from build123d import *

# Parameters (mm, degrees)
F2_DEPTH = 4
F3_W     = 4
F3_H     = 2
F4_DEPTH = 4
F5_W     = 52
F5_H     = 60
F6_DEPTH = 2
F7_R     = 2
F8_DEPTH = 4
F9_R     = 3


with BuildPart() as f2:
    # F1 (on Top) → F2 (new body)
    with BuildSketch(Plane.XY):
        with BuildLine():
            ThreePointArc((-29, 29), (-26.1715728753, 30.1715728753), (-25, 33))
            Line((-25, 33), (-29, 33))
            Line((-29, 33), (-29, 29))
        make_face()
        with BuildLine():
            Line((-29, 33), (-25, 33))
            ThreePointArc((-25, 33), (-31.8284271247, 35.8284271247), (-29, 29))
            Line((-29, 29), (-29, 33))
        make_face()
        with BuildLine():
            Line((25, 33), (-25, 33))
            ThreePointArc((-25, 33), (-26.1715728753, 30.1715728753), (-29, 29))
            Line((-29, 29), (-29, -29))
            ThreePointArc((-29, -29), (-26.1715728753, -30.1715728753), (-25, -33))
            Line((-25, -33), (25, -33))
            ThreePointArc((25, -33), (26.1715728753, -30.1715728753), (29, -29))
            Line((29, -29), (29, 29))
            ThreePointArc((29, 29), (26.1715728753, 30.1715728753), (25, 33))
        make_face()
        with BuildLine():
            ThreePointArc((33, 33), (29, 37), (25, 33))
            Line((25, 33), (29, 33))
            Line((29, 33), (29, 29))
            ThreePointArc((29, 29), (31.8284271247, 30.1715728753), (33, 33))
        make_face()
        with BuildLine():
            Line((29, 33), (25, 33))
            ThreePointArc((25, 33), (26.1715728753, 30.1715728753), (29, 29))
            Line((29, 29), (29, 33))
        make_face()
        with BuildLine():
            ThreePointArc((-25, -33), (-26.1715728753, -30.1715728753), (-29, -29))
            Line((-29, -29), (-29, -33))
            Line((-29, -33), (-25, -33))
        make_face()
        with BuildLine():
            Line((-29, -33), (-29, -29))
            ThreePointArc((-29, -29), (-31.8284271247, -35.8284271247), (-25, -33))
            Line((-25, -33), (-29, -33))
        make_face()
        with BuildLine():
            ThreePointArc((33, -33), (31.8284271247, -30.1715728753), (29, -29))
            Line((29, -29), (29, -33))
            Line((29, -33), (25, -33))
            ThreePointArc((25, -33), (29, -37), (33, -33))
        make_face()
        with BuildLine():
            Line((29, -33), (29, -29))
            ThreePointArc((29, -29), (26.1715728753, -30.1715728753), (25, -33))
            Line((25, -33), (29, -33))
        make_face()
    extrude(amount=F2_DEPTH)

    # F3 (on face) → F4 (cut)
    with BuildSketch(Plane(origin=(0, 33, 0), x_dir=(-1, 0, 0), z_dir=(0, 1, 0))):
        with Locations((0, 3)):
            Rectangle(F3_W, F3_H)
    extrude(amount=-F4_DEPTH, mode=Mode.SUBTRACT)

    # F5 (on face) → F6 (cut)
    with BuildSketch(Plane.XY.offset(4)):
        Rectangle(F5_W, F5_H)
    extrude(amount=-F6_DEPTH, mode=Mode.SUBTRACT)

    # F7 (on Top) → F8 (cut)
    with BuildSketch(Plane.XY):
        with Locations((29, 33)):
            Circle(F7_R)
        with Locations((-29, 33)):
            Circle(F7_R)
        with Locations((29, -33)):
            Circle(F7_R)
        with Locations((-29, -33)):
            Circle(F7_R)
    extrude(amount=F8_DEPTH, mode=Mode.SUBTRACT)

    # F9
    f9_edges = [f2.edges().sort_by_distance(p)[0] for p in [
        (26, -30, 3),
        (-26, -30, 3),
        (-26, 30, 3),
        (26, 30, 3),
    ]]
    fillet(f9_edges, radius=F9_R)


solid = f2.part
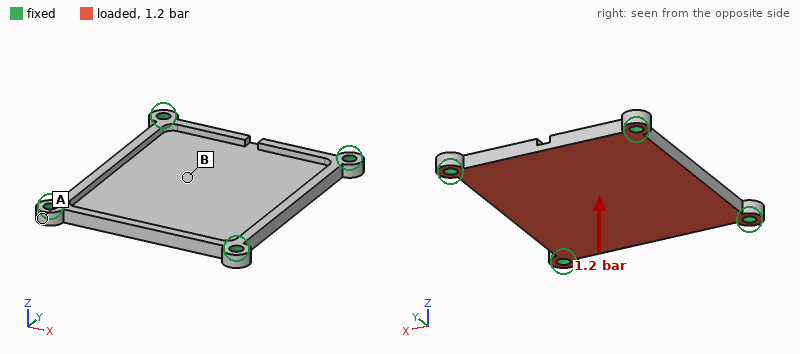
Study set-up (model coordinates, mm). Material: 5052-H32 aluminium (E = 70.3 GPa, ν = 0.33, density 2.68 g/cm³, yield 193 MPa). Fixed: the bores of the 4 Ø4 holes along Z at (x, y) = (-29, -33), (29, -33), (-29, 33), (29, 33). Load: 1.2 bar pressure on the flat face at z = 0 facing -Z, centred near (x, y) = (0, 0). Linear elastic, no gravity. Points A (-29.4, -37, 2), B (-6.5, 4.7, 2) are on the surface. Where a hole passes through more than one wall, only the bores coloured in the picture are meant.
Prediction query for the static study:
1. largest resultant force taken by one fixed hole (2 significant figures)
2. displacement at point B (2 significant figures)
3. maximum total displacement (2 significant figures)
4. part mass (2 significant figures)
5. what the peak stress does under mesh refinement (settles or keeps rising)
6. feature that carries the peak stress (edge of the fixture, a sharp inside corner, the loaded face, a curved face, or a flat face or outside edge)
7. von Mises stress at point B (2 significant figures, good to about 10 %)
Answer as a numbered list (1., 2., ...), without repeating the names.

1. 220 N
2. 0.12 mm
3. 0.13 mm
4. 25 g
5. keeps rising
6. edge of the fixture
7. 23 MPa
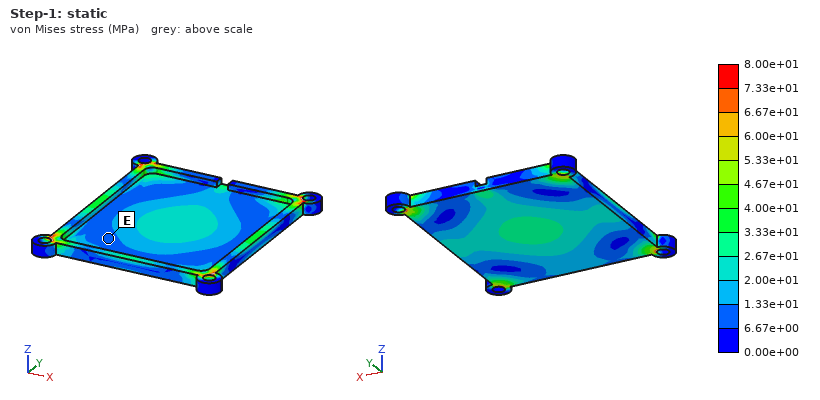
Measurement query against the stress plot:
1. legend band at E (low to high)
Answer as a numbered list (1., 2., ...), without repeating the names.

1. 6.67e+00 to 1.33e+01 MPa
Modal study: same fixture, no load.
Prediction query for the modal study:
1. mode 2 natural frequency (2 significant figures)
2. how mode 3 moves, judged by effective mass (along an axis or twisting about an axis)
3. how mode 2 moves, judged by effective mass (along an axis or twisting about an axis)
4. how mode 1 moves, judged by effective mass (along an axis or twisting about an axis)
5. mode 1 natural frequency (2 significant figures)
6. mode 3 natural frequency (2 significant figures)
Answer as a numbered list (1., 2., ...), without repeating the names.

1. 4400 Hz
2. twisting about X
3. twisting about Y
4. along Z
5. 2600 Hz
6. 4900 Hz
